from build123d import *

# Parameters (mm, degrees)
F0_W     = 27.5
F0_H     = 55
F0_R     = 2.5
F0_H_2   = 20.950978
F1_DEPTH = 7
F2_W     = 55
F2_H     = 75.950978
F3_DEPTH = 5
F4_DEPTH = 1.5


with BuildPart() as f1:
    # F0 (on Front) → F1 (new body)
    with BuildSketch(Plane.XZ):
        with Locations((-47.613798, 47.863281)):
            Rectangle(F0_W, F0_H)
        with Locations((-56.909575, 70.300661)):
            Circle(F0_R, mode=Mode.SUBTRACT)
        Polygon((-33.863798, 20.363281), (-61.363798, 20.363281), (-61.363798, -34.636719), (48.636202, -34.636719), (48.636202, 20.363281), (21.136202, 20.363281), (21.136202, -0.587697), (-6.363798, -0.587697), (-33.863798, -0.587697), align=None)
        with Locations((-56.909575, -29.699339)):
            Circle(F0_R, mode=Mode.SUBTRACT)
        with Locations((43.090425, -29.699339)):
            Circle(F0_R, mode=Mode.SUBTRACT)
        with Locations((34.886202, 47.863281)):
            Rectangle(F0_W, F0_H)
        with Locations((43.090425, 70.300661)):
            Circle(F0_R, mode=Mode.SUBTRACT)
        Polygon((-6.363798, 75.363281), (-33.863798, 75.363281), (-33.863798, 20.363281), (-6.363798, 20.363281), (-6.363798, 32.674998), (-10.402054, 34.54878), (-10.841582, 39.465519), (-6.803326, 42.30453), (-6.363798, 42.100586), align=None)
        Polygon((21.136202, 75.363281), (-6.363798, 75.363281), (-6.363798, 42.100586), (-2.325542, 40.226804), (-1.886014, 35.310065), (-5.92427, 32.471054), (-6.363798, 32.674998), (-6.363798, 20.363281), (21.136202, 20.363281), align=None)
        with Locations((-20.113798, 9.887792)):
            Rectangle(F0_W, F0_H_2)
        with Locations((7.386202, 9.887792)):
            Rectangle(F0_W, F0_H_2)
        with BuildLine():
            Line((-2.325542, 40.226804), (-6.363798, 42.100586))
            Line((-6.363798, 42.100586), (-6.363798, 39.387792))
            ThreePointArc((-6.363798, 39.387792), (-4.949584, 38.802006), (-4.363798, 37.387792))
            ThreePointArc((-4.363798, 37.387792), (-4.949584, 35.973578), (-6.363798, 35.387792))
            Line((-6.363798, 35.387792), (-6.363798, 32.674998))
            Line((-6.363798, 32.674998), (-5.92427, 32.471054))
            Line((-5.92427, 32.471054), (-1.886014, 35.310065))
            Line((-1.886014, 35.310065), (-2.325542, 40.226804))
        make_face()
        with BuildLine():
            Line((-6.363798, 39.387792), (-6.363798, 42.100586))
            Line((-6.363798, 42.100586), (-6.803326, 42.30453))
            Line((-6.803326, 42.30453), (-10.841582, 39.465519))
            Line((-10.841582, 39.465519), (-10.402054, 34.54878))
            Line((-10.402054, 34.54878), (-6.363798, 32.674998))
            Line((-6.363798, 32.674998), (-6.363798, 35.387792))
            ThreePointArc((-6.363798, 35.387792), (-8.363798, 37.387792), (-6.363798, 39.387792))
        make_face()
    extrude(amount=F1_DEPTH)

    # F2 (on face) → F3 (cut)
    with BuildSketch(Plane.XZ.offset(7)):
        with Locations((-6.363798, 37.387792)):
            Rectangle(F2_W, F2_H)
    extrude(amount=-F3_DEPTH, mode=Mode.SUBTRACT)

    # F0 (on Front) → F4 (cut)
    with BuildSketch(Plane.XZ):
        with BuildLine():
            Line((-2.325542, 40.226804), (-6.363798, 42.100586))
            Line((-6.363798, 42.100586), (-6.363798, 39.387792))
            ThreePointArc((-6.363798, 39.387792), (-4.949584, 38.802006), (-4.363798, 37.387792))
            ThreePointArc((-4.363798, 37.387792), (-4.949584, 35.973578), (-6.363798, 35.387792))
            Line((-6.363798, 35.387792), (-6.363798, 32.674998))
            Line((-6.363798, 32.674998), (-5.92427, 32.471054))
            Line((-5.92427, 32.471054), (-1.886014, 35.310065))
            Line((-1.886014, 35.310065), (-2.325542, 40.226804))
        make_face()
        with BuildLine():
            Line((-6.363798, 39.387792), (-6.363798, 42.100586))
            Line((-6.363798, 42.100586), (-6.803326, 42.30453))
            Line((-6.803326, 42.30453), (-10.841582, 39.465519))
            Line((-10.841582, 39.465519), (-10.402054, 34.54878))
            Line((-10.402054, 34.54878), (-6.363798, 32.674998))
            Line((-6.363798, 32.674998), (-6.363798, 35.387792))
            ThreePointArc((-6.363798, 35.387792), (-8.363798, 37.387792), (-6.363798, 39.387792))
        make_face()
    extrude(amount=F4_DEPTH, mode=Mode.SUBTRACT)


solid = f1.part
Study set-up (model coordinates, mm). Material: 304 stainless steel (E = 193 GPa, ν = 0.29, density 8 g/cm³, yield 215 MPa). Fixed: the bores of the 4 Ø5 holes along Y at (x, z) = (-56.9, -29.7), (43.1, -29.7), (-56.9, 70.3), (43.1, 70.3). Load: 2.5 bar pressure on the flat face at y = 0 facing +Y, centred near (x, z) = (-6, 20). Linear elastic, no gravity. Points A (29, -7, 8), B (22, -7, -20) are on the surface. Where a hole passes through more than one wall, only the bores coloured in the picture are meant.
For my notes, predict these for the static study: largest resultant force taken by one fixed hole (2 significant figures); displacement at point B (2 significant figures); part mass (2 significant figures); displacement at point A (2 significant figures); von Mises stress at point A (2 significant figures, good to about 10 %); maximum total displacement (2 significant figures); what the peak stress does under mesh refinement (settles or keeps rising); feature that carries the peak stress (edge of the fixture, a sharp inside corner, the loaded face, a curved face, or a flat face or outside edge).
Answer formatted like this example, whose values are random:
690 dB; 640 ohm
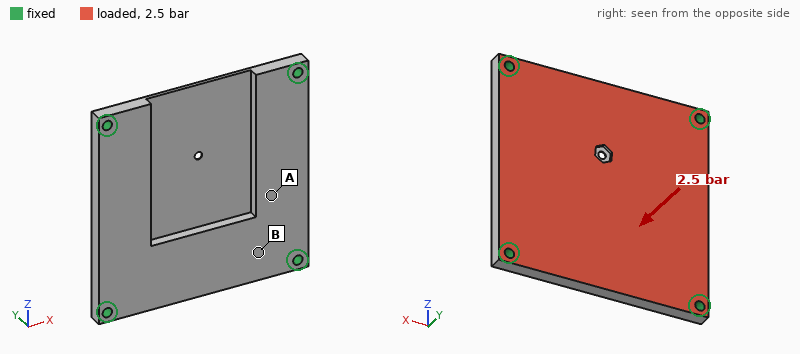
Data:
1.4 kN; 0.020 mm; 510 g; 0.035 mm; 24 MPa; 0.10 mm; keeps rising; edge of the fixture
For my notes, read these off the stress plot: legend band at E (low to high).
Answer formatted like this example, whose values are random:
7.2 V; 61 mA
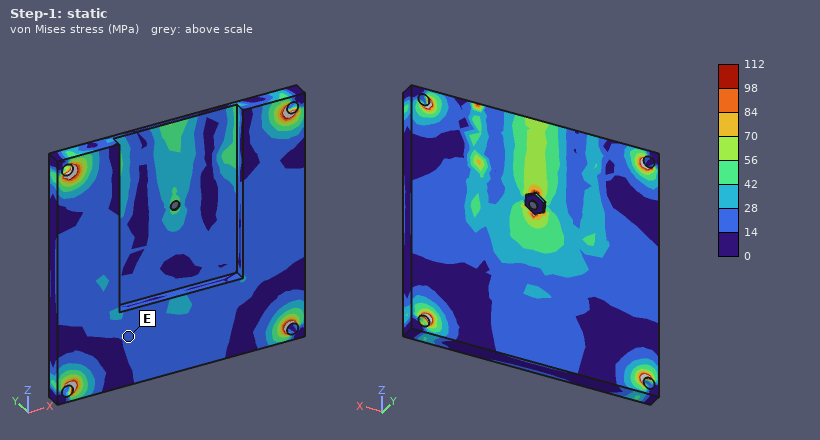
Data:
14 to 28 MPa
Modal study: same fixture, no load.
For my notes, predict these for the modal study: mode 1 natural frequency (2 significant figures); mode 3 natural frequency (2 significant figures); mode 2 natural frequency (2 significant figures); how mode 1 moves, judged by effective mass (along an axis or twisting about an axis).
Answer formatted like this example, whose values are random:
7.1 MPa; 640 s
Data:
2200 Hz; 3200 Hz; 3100 Hz; along Y
